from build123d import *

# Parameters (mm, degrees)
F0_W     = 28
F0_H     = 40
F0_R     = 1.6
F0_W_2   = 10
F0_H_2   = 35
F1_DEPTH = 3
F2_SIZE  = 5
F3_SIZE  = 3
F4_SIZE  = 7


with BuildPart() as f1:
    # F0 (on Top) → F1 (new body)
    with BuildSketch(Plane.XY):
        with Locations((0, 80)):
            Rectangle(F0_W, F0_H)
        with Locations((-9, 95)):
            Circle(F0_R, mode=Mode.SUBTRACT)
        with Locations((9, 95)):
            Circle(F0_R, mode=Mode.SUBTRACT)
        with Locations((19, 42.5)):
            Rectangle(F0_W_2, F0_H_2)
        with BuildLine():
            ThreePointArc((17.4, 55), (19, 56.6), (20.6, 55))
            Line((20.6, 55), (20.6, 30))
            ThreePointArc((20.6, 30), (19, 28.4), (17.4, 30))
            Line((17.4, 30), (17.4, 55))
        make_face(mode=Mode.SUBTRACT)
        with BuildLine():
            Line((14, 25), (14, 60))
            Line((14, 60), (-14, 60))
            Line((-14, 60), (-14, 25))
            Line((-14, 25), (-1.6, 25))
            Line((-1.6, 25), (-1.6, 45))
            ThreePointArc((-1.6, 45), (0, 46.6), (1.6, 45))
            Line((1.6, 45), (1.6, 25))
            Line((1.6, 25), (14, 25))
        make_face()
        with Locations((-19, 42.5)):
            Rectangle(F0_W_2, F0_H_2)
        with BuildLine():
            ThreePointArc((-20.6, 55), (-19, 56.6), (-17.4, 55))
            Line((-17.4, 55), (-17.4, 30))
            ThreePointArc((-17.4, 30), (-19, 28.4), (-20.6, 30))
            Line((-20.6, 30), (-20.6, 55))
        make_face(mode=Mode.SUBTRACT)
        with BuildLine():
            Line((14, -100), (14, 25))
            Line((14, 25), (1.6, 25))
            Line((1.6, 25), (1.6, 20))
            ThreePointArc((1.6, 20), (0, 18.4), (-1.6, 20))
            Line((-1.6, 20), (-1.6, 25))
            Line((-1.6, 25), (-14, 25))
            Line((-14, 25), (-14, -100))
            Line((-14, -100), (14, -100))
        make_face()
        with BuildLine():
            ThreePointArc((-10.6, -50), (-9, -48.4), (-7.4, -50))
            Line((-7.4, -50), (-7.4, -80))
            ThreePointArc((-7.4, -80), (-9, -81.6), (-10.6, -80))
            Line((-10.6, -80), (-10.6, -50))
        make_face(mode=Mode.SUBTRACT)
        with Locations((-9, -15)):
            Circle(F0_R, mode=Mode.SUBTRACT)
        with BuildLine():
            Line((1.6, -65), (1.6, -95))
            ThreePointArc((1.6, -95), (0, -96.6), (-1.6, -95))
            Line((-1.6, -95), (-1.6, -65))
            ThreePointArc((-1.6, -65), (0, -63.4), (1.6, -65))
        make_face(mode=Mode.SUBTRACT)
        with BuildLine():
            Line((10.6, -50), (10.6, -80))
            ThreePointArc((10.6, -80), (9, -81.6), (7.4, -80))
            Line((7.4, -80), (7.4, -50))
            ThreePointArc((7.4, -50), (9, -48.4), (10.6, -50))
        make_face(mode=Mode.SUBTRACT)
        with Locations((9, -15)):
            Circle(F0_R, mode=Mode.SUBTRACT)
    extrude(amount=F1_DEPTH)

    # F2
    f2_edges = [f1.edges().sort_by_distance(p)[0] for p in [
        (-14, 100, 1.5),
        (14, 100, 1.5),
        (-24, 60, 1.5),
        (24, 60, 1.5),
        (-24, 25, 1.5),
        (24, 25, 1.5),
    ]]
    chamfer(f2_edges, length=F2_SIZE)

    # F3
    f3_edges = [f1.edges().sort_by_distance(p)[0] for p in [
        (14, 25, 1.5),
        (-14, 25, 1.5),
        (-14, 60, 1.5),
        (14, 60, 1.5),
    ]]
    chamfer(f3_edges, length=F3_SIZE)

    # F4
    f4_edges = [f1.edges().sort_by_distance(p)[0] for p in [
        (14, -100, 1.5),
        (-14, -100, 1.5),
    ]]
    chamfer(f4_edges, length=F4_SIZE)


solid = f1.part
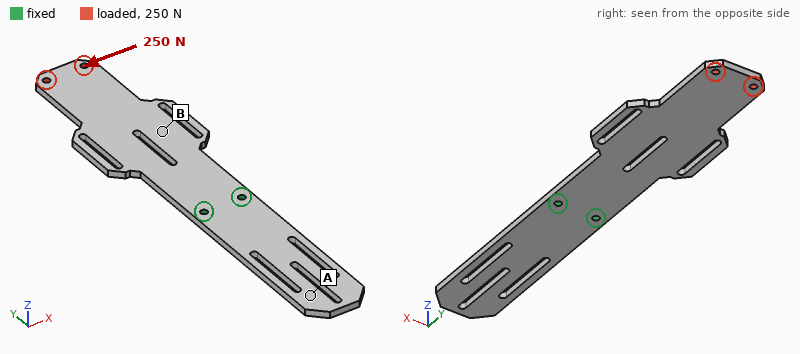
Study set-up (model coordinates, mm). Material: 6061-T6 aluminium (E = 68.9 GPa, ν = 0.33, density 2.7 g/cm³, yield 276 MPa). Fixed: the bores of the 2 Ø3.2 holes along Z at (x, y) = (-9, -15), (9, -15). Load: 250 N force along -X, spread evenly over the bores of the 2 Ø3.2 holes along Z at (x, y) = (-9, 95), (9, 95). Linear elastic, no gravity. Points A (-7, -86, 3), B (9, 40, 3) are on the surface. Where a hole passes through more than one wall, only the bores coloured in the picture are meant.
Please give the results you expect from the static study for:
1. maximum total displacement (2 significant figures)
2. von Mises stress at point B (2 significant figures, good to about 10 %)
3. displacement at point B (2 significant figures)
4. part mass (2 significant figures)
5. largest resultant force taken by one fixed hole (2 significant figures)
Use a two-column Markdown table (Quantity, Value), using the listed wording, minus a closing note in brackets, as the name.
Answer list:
| Quantity | Value |
|---|---|
| maximum total displacement | 0.32 mm |
| von Mises stress at point B | 16 MPa |
| displacement at point B | 0.12 mm |
| part mass | 45 g |
| largest resultant force taken by one fixed hole | 1.4 kN |
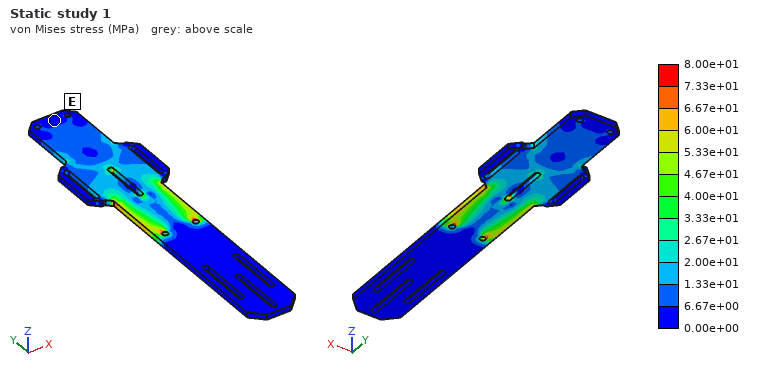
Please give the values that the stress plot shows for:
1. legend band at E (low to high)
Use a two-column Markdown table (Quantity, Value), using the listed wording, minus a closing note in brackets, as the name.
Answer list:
| Quantity | Value |
|---|---|
| legend band at E | 0.00e+00 to 6.67e+00 MPa |
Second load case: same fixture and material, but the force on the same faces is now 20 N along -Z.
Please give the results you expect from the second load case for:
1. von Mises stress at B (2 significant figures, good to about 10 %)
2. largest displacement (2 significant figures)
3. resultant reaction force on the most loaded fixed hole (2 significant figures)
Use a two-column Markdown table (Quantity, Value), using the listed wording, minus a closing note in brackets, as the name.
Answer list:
| Quantity | Value |
|---|---|
| von Mises stress at B | 21 MPa |
| largest displacement | 2.1 mm |
| resultant reaction force on the most loaded fixed hole | 10 N |
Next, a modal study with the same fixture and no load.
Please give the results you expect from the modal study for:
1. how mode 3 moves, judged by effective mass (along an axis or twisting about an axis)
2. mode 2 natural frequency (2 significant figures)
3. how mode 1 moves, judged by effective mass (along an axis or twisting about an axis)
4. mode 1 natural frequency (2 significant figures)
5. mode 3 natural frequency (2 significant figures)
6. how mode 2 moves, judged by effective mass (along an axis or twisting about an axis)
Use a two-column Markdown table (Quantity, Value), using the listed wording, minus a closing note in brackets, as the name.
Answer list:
| Quantity | Value |
|---|---|
| how mode 3 moves, judged by effective mass | twisting about Y |
| mode 2 natural frequency | 380 Hz |
| how mode 1 moves, judged by effective mass | along Z |
| mode 1 natural frequency | 190 Hz |
| mode 3 natural frequency | 1100 Hz |
| how mode 2 moves, judged by effective mass | along Z |
